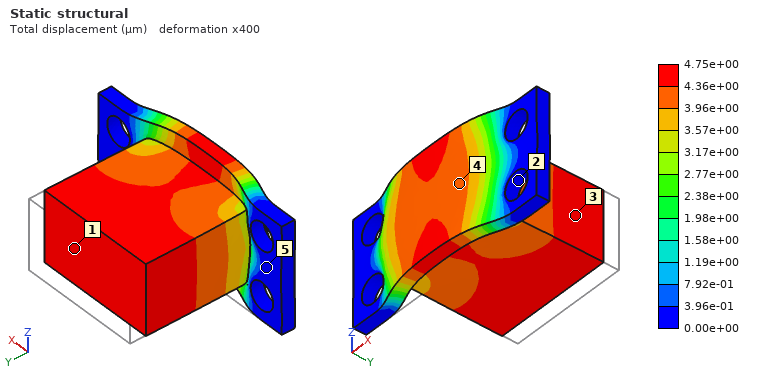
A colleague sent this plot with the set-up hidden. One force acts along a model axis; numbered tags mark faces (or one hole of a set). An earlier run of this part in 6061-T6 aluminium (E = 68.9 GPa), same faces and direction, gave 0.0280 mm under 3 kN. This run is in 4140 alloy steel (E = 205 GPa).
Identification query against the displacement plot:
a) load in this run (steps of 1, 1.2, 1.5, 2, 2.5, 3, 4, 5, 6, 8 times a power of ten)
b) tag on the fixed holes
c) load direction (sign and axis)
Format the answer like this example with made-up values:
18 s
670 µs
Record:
1.5 kN
2
-Y
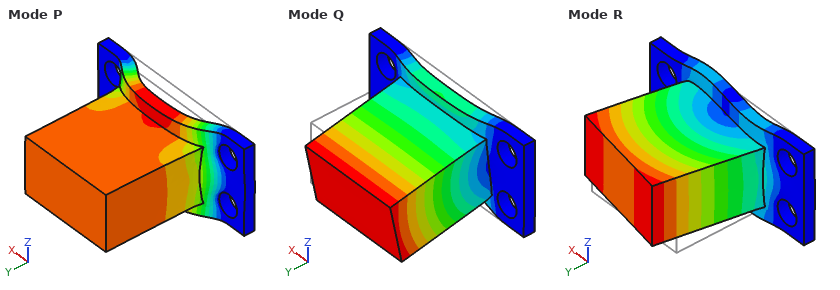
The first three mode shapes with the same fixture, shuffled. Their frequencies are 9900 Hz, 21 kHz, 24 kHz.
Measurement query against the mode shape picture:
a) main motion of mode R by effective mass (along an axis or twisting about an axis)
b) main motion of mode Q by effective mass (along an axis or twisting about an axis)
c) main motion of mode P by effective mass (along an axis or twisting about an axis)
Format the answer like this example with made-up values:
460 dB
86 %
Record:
along X
along Z
along Y
